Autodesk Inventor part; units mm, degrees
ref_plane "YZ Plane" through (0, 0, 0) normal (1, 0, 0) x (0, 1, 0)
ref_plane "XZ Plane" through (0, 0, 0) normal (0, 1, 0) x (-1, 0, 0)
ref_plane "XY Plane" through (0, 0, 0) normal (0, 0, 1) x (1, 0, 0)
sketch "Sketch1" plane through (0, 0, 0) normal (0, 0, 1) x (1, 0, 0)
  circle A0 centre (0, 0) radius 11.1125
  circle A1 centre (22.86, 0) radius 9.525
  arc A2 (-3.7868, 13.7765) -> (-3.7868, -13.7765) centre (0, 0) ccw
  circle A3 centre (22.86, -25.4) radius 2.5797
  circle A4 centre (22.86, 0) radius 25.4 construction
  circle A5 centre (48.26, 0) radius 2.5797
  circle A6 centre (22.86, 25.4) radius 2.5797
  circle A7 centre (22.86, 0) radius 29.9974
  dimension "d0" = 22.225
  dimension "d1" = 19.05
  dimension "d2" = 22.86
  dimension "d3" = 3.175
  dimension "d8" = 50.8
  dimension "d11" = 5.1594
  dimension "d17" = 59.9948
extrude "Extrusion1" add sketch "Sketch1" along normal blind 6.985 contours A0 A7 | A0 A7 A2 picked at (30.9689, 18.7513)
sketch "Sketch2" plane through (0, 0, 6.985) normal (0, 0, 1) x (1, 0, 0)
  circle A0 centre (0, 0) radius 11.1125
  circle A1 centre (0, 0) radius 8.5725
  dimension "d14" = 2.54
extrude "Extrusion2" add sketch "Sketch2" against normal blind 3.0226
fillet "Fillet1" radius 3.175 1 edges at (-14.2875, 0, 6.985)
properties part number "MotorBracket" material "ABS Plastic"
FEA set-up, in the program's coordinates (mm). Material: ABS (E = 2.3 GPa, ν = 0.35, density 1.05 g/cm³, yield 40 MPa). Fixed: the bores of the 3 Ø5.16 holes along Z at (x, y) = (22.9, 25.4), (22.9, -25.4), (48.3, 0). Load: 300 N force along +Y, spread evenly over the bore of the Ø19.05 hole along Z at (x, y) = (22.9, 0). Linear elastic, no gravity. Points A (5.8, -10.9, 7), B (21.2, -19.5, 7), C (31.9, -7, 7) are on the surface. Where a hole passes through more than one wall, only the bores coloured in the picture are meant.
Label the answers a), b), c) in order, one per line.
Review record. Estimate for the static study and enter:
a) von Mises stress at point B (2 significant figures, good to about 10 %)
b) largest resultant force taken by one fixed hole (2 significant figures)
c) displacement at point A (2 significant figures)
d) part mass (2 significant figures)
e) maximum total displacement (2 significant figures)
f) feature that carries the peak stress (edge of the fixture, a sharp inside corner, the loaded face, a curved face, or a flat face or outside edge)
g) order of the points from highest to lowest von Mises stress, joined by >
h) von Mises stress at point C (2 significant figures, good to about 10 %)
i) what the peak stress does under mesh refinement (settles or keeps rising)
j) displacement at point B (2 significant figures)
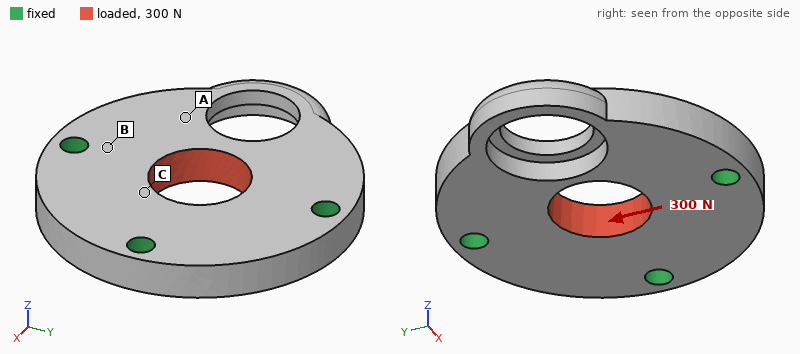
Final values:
a) 1.5 MPa
b) 120 N
c) 11 µm
d) 17 g
e) 14 µm
f) edge of the fixture
g) B > C > A
h) 0.86 MPa
i) keeps rising
j) 2.9 µm
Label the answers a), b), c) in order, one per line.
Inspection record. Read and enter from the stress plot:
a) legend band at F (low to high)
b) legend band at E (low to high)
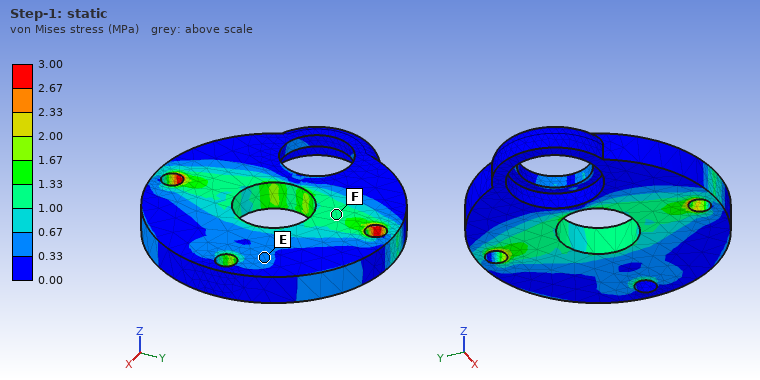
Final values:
a) 1.00 to 1.33 MPa
b) 0.33 to 0.67 MPa
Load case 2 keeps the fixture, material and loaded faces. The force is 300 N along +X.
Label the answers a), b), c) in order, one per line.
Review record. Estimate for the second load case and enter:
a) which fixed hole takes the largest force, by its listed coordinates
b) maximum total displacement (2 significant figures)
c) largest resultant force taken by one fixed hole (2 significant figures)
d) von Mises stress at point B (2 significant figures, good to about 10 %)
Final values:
a) (48.3, 0)
b) 36 µm
c) 130 N
d) 1.1 MPa
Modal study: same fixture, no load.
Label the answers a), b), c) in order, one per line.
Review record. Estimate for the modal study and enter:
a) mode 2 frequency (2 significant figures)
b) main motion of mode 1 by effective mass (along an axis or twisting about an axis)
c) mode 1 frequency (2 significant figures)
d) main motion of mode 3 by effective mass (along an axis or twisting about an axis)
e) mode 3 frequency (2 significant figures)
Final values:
a) 3400 Hz
b) along Z
c) 1600 Hz
d) along Z
e) 4500 Hz
